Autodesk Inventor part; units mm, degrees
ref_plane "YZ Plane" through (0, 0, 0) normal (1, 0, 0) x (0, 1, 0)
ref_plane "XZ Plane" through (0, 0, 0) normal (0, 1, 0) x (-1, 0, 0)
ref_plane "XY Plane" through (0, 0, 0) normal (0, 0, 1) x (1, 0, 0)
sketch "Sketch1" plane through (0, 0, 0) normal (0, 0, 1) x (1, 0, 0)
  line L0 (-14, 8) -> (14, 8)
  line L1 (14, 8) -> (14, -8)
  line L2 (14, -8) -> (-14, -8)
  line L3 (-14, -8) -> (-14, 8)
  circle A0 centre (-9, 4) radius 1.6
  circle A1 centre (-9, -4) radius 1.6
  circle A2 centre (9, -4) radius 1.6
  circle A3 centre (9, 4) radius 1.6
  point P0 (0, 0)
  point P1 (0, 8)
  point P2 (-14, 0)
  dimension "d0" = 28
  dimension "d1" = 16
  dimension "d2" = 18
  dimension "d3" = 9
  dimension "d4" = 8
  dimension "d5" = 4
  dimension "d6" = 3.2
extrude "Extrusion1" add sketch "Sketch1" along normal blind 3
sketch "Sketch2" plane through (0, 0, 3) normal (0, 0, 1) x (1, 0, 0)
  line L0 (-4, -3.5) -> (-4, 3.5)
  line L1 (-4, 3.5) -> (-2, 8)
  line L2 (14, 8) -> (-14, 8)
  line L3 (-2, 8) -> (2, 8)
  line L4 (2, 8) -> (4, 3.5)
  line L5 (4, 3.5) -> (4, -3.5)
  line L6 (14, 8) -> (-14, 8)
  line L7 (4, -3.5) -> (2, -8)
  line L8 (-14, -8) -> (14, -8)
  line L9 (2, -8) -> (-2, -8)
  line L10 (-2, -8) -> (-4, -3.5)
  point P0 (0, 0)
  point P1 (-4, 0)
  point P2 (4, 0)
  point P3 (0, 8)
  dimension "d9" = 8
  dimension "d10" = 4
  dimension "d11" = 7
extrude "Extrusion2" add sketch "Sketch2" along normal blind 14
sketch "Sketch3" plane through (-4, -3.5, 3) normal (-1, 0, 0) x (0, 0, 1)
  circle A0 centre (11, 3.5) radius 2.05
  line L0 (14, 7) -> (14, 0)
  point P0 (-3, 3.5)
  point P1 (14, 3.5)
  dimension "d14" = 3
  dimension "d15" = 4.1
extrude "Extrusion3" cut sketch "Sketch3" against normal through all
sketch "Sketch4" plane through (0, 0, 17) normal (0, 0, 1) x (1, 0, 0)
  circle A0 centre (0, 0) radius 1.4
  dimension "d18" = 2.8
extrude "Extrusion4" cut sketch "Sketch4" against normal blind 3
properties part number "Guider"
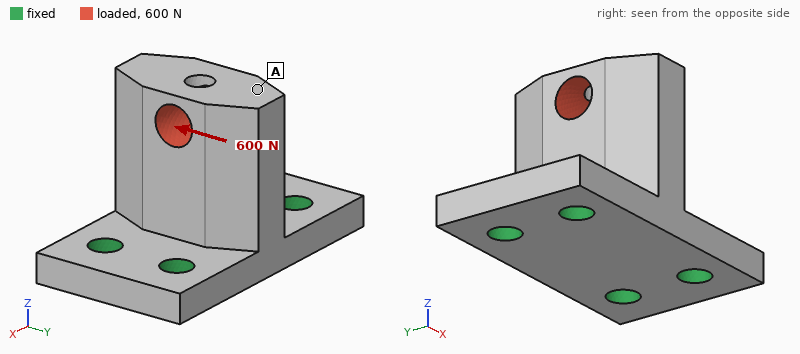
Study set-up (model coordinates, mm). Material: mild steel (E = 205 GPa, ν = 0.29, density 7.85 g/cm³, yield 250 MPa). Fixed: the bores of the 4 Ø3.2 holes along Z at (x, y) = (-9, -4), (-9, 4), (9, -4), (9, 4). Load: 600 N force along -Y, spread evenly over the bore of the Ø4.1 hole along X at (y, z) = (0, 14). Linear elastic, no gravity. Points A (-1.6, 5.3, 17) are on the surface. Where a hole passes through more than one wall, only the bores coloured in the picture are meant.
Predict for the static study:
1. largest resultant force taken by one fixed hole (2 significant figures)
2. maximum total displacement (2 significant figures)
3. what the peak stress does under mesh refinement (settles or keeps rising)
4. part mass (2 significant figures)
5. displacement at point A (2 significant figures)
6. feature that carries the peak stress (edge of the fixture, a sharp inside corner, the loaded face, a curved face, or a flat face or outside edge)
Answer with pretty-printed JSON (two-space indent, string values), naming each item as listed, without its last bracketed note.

{
  "largest resultant force taken by one fixed hole": "410 N",
  "maximum total displacement": "14 µm",
  "what the peak stress does under mesh refinement": "keeps rising",
  "part mass": "21 g",
  "displacement at point A": "13 µm",
  "feature that carries the peak stress": "edge of the fixture"
}
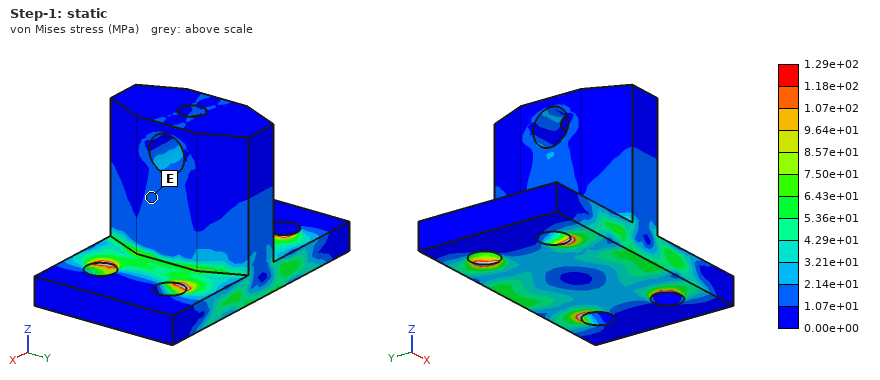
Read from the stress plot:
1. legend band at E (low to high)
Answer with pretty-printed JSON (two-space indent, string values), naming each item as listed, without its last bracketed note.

{
  "legend band at E": "1.07e+01 to 2.14e+01 MPa"
}
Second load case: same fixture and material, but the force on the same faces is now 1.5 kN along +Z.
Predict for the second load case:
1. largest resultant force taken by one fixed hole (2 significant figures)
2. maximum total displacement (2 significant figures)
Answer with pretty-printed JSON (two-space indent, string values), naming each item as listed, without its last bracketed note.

{
  "largest resultant force taken by one fixed hole": "390 N",
  "maximum total displacement": "5.1 µm"
}
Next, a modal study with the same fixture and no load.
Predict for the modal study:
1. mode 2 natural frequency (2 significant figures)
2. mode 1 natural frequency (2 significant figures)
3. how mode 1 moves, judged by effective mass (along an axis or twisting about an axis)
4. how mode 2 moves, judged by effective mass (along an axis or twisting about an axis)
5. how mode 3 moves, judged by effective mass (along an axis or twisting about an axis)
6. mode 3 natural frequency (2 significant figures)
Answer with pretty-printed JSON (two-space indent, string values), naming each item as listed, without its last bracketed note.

{
  "mode 2 natural frequency": "17 kHz",
  "mode 1 natural frequency": "14 kHz",
  "how mode 1 moves, judged by effective mass": "along Y",
  "how mode 2 moves, judged by effective mass": "along X",
  "how mode 3 moves, judged by effective mass": "along Z",
  "mode 3 natural frequency": "29 kHz"
}
